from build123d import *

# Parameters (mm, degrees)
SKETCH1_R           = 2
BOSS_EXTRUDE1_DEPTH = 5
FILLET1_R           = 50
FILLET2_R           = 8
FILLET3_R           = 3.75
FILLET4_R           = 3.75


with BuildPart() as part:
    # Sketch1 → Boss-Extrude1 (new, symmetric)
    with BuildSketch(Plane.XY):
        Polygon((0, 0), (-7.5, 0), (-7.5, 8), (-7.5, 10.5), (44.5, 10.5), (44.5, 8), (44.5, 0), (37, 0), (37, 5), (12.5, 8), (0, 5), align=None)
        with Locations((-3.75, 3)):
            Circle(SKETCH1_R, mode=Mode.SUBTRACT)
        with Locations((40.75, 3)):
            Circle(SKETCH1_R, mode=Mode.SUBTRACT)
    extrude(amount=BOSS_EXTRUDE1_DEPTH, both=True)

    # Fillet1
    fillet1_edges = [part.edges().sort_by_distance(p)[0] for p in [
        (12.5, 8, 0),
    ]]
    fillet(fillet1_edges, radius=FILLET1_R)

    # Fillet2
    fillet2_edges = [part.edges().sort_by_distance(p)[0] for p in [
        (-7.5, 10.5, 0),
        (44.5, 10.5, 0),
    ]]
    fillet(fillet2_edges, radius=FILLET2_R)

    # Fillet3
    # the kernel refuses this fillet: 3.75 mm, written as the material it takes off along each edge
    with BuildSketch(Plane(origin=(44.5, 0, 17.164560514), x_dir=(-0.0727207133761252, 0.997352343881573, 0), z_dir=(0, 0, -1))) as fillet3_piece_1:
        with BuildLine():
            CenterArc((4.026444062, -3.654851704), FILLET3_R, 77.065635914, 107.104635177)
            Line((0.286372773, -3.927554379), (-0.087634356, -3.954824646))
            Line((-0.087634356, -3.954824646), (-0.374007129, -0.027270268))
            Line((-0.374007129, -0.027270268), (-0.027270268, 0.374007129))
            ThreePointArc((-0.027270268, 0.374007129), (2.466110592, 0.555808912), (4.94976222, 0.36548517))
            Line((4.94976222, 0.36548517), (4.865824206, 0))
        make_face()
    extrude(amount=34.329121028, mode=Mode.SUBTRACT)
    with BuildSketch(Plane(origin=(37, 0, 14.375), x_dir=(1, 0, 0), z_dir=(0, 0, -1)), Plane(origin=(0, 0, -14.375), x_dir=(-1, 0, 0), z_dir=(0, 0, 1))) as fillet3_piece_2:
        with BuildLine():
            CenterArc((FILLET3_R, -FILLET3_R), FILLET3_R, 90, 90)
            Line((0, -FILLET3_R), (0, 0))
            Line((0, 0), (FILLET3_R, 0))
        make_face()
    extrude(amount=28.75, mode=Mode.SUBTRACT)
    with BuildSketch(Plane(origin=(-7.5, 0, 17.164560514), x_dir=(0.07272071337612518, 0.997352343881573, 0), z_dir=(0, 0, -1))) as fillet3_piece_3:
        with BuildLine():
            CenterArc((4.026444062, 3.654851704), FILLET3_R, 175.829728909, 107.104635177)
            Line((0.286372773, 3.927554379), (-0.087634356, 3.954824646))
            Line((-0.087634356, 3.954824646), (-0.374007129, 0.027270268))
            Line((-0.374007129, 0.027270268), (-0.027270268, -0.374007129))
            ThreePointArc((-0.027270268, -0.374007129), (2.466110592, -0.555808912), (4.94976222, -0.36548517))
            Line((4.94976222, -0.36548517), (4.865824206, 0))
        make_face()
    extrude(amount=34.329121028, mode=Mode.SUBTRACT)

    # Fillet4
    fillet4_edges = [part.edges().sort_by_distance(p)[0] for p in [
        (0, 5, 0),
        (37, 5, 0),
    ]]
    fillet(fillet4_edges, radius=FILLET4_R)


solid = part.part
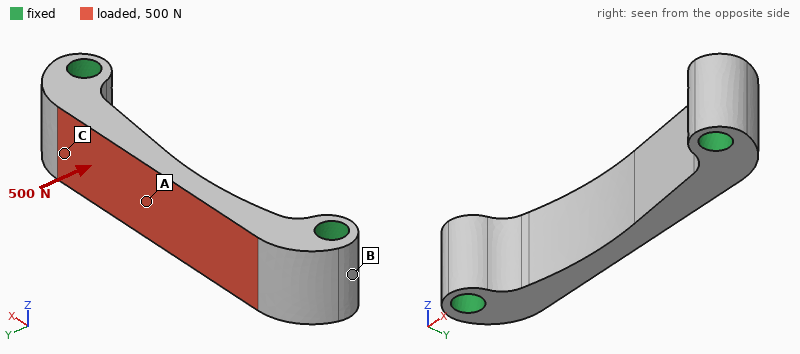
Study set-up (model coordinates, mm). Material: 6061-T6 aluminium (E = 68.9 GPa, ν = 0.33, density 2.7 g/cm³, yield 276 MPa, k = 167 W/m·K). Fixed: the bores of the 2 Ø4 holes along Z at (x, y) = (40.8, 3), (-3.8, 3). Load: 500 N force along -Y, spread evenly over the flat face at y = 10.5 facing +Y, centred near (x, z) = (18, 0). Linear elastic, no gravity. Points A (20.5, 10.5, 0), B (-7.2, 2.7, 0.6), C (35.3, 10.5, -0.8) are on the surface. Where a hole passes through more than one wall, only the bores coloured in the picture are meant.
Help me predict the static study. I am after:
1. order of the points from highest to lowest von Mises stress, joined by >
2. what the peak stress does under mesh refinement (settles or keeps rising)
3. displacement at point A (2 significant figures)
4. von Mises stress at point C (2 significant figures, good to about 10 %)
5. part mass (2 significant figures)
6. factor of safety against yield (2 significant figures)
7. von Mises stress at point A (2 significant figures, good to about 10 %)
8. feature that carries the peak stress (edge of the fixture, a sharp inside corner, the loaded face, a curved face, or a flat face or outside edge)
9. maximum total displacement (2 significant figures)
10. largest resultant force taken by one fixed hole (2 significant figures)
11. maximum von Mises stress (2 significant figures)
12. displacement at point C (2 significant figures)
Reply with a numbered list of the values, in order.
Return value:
1. A > C > B
2. settles
3. 18 µm
4. 16 MPa
5. 6.7 g
6. 6.3
7. 31 MPa
8. a curved face
9. 20 µm
10. 390 N
11. 44 MPa
12. 3.6 µm
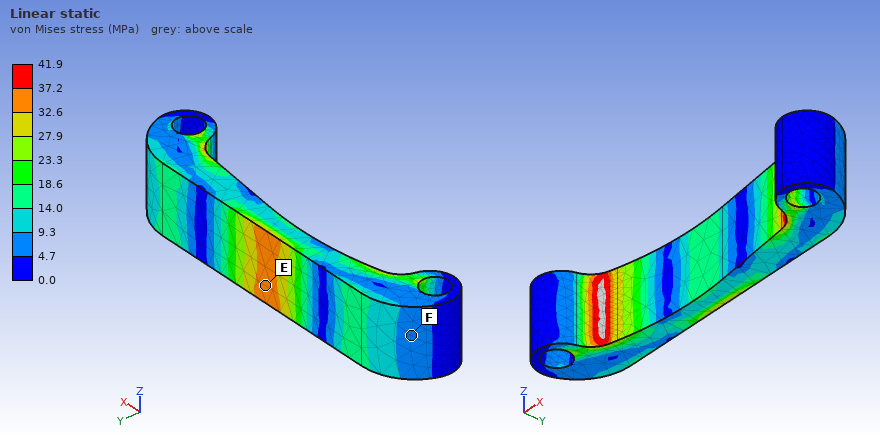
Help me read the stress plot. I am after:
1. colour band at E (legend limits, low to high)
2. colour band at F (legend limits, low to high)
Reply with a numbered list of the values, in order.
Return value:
1. 32.6 to 37.2 MPa
2. 4.7 to 9.3 MPa
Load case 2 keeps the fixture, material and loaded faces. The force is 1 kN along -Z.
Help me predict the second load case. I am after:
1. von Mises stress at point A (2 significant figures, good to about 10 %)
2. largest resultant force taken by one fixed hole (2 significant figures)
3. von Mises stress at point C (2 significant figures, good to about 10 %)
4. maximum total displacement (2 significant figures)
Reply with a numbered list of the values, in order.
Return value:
1. 13 MPa
2. 500 N
3. 33 MPa
4. 24 µm
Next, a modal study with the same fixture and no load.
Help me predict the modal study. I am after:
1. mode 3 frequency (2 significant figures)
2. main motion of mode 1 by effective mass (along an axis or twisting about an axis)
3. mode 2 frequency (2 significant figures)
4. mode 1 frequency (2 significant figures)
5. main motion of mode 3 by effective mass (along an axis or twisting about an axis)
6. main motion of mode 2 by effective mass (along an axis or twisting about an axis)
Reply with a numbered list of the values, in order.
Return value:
1. 29 kHz
2. along Y
3. 22 kHz
4. 16 kHz
5. along X
6. along Z
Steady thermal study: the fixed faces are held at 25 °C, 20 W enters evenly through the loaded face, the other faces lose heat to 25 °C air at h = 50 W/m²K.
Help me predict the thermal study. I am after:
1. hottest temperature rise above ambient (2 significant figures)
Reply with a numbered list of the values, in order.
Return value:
1. 17 K
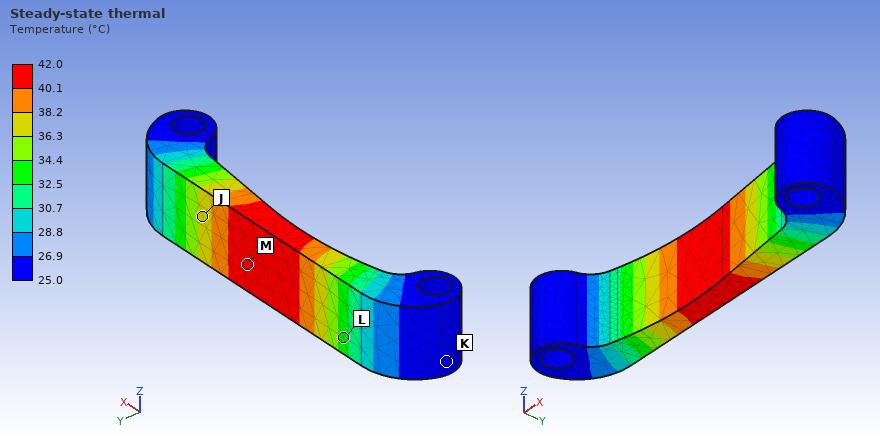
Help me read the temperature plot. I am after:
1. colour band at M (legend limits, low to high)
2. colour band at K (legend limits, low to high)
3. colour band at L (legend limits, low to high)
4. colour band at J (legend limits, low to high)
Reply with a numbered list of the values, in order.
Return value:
1. 40.1 to 42.0 °C
2. 25.0 to 26.9 °C
3. 32.5 to 34.4 °C
4. 36.3 to 38.2 °C
